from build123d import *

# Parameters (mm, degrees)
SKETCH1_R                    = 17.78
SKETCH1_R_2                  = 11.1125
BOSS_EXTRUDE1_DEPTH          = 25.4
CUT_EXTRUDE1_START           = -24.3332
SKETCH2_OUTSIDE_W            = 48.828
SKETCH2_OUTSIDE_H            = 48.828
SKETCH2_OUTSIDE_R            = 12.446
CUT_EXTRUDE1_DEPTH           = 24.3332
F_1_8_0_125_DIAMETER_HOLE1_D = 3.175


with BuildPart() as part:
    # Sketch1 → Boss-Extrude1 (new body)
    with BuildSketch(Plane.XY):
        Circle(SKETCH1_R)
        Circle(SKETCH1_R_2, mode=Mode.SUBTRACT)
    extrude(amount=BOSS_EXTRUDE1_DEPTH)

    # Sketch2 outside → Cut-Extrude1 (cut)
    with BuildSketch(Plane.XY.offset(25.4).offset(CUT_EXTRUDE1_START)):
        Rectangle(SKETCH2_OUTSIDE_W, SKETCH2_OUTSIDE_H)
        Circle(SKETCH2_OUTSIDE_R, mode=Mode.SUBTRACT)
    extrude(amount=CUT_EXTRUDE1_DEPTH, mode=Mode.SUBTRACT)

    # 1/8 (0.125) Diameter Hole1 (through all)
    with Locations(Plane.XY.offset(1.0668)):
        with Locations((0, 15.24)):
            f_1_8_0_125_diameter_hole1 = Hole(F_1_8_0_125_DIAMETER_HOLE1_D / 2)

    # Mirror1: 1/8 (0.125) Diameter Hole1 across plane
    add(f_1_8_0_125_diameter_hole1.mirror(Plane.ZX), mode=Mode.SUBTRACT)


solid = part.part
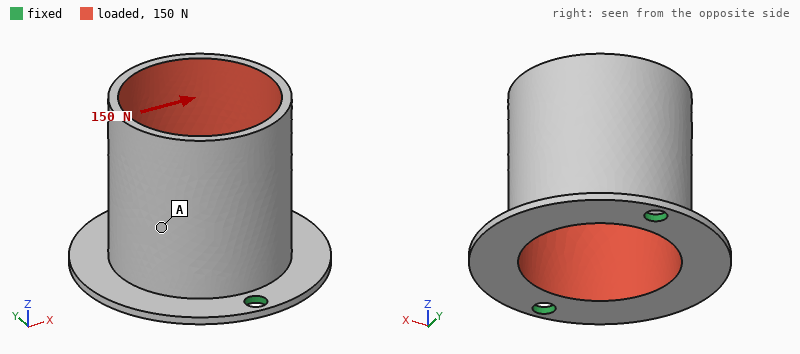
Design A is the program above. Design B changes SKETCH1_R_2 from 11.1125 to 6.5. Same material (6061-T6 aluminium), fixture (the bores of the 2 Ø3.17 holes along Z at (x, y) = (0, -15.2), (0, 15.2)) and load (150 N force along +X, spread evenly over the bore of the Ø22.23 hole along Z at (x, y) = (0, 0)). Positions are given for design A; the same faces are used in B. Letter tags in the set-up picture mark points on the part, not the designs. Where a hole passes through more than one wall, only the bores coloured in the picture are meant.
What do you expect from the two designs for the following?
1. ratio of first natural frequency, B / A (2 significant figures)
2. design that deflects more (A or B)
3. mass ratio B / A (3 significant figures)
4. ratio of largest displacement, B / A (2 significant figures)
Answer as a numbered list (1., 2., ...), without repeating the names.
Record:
1. 0.61
2. A
3. 3.14
4. 0.87
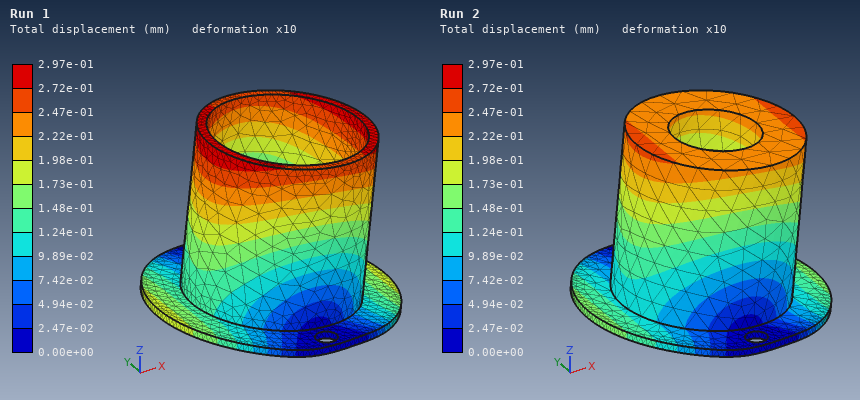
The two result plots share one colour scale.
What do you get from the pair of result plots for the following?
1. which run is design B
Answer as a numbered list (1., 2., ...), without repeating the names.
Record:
1. Run 2
